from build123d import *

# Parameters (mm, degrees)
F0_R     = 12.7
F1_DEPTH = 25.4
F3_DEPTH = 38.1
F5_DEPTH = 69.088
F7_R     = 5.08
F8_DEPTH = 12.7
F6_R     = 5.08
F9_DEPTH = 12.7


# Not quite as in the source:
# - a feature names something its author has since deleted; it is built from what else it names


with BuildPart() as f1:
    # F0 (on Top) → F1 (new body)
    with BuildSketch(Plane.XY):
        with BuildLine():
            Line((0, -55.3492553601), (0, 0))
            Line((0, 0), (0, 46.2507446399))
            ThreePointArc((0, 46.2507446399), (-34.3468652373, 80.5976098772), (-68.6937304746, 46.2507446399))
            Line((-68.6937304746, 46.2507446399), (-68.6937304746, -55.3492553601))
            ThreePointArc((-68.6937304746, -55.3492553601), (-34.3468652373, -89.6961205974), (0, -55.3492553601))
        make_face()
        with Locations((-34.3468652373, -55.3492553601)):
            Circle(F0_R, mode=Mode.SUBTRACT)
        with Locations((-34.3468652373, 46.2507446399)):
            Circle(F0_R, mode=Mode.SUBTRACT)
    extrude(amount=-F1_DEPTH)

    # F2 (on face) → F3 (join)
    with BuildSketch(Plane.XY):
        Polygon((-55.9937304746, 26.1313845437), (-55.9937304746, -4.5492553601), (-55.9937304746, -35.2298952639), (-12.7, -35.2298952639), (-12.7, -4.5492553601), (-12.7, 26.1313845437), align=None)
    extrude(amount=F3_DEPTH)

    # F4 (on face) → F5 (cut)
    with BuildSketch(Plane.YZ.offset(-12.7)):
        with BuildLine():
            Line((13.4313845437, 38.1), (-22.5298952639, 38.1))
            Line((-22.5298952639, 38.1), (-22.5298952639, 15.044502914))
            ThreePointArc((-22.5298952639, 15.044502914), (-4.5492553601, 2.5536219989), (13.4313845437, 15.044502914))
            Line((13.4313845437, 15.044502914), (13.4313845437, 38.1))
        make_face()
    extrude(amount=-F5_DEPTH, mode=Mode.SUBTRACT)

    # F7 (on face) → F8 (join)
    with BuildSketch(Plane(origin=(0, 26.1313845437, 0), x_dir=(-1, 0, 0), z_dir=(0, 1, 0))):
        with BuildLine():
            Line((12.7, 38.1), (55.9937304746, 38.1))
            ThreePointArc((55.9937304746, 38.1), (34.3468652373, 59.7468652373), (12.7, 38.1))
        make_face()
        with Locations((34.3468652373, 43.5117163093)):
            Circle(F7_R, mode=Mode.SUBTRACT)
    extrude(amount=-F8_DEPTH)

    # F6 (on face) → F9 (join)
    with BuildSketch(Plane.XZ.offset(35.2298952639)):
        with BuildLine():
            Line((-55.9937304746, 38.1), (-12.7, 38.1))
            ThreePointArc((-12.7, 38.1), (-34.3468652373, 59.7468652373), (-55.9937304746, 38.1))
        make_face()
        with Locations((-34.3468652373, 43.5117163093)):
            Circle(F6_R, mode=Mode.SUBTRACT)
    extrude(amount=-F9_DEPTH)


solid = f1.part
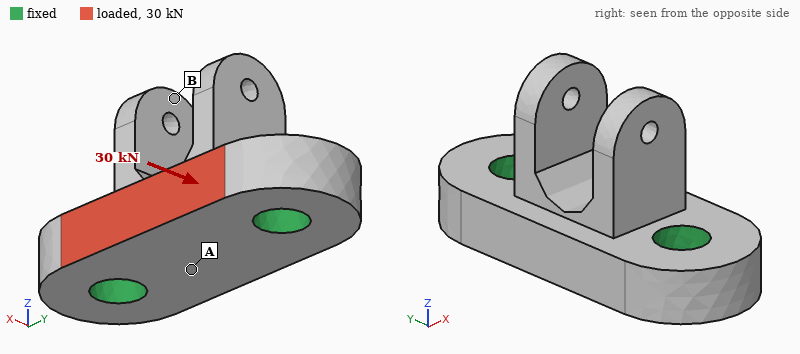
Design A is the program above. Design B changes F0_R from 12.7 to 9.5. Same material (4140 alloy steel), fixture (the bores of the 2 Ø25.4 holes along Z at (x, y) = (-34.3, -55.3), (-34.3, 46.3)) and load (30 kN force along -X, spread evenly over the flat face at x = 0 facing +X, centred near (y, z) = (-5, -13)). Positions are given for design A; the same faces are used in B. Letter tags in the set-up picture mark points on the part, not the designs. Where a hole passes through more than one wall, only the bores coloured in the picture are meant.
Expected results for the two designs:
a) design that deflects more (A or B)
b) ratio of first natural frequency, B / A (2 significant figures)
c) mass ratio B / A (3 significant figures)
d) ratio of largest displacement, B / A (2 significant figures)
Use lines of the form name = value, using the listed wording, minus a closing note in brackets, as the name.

design that deflects more = B
ratio of first natural frequency, B / A = 0.99
mass ratio B / A = 1.04
ratio of largest displacement, B / A = 1.2
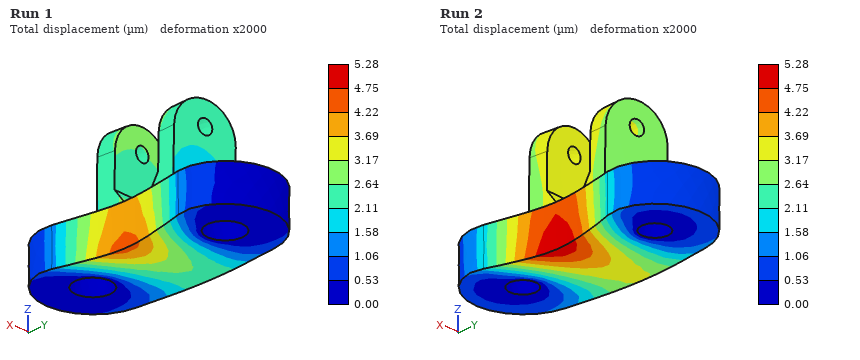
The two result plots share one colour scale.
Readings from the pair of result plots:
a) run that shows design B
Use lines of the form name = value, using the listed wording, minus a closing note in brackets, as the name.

run that shows design B = Run 2
